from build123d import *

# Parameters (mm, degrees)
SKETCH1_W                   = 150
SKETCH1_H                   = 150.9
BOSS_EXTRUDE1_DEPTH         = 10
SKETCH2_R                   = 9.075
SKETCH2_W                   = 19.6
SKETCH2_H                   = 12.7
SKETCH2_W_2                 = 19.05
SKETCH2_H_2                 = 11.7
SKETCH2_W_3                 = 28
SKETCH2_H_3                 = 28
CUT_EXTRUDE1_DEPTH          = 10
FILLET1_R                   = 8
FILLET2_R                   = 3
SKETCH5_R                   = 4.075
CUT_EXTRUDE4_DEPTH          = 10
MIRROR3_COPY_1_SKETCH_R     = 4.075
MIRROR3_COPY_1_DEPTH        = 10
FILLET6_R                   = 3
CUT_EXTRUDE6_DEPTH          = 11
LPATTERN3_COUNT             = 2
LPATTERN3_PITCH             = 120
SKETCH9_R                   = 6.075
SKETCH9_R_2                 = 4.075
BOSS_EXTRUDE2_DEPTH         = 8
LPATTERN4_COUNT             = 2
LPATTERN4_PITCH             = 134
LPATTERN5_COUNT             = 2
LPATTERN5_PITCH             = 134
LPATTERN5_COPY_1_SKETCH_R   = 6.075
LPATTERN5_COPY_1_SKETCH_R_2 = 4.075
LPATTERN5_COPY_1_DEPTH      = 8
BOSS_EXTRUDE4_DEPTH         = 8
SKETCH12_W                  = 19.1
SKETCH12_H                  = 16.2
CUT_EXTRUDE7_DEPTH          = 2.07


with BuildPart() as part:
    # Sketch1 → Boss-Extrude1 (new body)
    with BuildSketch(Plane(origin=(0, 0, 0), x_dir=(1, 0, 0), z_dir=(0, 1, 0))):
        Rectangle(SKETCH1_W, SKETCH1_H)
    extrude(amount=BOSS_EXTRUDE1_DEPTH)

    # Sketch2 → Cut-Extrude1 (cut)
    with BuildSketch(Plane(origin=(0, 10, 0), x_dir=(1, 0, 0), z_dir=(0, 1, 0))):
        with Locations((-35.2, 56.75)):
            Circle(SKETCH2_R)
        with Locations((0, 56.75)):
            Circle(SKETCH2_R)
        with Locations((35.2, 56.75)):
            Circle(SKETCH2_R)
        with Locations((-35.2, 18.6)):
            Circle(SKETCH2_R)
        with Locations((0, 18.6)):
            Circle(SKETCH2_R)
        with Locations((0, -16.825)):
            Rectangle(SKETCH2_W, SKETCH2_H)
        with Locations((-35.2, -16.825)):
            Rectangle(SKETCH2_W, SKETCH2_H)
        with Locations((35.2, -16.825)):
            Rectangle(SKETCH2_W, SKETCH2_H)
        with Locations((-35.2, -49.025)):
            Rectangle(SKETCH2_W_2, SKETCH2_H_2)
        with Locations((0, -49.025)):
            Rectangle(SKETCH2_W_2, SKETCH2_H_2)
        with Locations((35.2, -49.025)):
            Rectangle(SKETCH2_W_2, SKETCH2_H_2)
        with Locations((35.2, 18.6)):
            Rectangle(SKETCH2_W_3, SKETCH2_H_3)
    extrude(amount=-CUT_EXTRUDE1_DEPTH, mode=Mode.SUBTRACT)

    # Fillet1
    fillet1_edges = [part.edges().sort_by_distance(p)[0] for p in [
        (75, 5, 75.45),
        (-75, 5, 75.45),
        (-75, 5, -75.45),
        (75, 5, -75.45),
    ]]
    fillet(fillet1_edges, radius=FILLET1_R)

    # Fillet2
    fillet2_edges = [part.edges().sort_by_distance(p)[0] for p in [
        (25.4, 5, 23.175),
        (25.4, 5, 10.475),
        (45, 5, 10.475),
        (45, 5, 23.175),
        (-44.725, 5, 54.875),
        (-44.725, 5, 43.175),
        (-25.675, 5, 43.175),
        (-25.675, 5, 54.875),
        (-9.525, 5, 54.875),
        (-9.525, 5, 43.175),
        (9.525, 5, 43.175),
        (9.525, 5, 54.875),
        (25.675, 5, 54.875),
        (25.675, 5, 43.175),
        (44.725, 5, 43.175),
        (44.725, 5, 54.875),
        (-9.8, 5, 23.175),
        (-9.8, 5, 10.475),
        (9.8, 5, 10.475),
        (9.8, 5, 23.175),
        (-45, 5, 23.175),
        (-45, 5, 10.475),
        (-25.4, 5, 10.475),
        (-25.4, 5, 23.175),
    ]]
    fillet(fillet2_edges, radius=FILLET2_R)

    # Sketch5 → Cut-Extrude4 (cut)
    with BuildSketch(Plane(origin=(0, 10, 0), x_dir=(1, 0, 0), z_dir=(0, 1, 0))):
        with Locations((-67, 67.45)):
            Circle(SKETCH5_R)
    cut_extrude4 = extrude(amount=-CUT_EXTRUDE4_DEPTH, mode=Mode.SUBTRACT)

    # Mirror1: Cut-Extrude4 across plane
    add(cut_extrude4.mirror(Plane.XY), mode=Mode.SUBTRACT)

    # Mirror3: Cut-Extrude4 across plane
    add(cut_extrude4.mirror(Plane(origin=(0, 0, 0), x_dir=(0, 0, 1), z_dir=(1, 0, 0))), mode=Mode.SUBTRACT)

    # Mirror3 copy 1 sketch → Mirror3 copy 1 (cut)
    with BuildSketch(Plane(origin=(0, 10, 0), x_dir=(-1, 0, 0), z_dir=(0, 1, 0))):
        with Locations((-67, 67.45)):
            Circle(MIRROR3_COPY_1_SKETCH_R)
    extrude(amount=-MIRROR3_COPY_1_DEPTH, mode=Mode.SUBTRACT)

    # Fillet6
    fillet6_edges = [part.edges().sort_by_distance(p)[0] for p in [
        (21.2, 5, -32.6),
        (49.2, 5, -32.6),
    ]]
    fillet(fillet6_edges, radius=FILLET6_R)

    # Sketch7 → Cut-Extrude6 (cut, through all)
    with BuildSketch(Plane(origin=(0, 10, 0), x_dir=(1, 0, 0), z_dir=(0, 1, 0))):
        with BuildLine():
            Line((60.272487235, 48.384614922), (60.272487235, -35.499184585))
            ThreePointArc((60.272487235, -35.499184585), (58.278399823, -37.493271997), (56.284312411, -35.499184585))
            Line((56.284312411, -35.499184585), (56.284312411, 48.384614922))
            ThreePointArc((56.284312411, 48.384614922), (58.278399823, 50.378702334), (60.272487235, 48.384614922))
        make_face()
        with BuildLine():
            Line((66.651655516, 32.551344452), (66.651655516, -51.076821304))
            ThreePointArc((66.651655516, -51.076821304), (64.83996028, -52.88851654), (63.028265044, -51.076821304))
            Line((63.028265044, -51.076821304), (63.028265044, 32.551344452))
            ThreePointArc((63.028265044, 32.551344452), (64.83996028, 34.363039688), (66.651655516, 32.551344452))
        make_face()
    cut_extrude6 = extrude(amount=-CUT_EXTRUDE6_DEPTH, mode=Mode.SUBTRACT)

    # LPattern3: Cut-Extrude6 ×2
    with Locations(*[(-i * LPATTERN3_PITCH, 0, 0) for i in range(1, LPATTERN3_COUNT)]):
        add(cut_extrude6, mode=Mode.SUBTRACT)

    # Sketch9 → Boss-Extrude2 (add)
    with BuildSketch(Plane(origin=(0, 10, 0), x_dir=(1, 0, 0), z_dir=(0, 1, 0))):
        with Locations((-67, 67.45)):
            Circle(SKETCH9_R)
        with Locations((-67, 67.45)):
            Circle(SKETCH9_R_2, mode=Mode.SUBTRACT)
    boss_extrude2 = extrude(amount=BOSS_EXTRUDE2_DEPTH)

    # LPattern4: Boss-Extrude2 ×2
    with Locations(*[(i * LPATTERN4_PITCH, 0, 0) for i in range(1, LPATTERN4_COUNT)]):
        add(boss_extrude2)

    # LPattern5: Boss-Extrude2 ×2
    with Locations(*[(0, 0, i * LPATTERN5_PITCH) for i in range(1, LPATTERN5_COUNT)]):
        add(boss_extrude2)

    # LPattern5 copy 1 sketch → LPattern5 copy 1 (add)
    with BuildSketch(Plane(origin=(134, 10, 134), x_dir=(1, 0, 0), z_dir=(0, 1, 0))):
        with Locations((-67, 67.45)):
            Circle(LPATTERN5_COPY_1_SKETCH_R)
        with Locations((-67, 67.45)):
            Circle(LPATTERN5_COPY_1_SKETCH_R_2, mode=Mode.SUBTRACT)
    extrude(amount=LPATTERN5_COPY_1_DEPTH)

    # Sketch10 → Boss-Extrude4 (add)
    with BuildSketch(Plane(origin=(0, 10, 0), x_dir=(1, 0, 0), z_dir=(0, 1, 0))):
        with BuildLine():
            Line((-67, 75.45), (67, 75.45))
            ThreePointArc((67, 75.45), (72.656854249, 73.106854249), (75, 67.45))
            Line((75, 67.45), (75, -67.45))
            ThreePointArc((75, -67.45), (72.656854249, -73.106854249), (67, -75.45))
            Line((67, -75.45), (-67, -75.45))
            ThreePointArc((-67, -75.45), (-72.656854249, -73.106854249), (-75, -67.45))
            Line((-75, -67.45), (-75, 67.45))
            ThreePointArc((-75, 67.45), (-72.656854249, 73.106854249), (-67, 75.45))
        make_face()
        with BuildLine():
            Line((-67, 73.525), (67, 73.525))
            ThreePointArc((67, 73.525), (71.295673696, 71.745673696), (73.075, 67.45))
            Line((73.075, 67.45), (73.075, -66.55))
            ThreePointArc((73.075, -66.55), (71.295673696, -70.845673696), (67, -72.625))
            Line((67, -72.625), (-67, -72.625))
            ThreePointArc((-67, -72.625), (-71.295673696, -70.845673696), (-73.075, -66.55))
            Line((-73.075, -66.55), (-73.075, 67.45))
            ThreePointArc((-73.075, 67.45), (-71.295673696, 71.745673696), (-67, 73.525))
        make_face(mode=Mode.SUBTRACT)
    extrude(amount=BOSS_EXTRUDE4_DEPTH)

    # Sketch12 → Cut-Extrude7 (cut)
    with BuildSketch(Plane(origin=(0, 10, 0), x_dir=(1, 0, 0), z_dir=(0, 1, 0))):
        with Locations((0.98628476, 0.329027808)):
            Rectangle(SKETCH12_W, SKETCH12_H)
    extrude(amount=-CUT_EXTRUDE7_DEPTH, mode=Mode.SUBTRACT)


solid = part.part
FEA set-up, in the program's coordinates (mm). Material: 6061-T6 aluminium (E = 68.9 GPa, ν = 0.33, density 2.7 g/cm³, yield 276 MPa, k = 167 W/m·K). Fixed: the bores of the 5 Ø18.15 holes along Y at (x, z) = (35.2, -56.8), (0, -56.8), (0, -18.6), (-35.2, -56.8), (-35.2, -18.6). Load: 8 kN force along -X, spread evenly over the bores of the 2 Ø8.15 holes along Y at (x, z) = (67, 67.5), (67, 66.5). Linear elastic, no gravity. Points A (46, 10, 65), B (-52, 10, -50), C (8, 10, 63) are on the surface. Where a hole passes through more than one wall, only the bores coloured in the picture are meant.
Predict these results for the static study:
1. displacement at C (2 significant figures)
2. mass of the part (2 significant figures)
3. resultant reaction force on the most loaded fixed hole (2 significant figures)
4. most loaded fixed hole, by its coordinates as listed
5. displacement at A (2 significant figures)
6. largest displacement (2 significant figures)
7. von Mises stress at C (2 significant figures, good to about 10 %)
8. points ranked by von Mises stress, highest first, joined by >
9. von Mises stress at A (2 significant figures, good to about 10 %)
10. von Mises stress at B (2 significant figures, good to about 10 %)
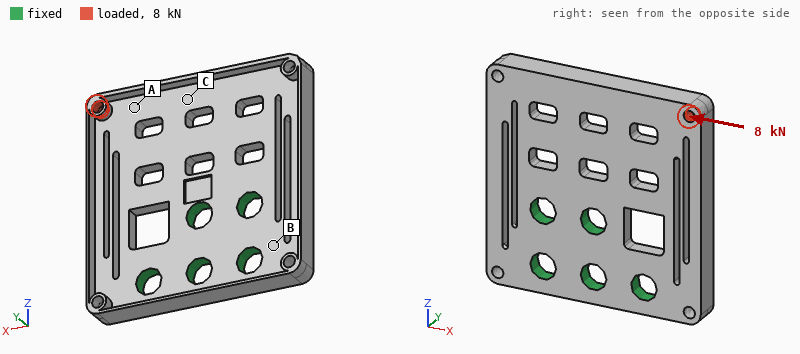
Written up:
0.11 mm
510 g
8.0 kN
(-35.2, -18.6)
0.21 mm
0.41 mm
38 MPa
A > C > B
53 MPa
10 MPa
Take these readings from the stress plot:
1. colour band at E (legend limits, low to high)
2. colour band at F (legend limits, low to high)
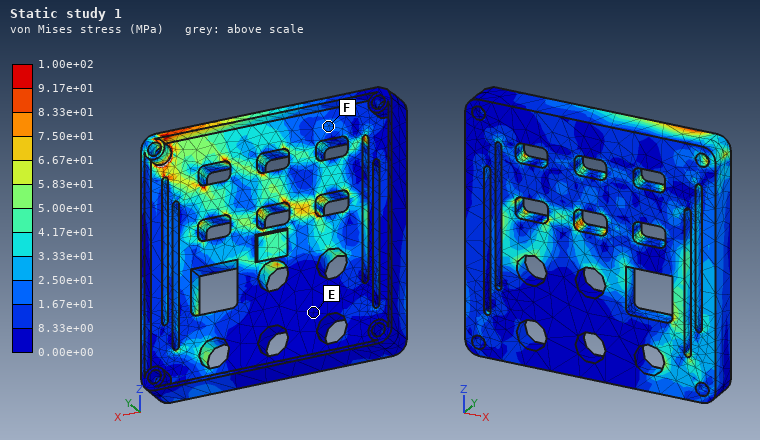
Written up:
0.00e+00 to 8.33e+00 MPa
1.67e+01 to 2.50e+01 MPa
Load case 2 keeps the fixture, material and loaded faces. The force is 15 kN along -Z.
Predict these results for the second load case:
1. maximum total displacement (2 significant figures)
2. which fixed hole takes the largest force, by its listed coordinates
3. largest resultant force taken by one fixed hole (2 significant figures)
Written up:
0.81 mm
(35.2, -56.8)
13 kN
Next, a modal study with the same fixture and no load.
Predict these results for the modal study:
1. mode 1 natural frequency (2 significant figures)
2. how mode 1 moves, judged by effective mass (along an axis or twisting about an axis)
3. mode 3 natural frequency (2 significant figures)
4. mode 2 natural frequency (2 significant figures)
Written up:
700 Hz
along Y
2400 Hz
1000 Hz
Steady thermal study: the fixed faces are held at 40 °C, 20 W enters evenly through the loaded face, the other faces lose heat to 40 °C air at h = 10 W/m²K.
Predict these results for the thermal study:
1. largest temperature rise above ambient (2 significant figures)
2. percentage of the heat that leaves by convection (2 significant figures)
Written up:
25 K
15 %
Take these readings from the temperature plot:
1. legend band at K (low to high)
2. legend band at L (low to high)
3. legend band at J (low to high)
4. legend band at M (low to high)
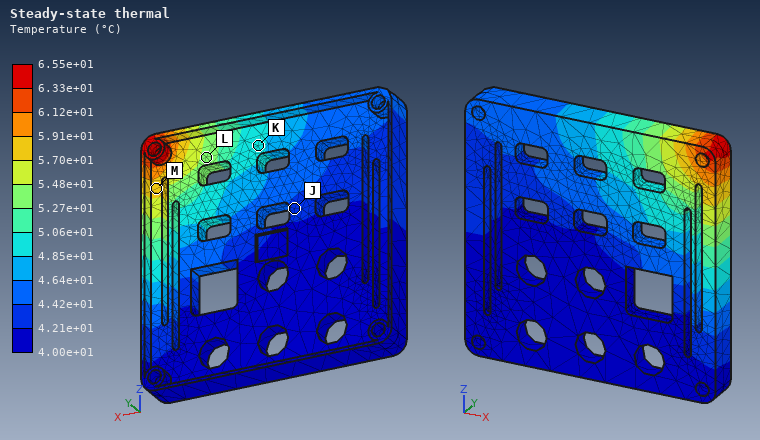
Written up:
4.85e+01 to 5.06e+01 °C
5.27e+01 to 5.48e+01 °C
4.21e+01 to 4.42e+01 °C
5.70e+01 to 5.91e+01 °C
